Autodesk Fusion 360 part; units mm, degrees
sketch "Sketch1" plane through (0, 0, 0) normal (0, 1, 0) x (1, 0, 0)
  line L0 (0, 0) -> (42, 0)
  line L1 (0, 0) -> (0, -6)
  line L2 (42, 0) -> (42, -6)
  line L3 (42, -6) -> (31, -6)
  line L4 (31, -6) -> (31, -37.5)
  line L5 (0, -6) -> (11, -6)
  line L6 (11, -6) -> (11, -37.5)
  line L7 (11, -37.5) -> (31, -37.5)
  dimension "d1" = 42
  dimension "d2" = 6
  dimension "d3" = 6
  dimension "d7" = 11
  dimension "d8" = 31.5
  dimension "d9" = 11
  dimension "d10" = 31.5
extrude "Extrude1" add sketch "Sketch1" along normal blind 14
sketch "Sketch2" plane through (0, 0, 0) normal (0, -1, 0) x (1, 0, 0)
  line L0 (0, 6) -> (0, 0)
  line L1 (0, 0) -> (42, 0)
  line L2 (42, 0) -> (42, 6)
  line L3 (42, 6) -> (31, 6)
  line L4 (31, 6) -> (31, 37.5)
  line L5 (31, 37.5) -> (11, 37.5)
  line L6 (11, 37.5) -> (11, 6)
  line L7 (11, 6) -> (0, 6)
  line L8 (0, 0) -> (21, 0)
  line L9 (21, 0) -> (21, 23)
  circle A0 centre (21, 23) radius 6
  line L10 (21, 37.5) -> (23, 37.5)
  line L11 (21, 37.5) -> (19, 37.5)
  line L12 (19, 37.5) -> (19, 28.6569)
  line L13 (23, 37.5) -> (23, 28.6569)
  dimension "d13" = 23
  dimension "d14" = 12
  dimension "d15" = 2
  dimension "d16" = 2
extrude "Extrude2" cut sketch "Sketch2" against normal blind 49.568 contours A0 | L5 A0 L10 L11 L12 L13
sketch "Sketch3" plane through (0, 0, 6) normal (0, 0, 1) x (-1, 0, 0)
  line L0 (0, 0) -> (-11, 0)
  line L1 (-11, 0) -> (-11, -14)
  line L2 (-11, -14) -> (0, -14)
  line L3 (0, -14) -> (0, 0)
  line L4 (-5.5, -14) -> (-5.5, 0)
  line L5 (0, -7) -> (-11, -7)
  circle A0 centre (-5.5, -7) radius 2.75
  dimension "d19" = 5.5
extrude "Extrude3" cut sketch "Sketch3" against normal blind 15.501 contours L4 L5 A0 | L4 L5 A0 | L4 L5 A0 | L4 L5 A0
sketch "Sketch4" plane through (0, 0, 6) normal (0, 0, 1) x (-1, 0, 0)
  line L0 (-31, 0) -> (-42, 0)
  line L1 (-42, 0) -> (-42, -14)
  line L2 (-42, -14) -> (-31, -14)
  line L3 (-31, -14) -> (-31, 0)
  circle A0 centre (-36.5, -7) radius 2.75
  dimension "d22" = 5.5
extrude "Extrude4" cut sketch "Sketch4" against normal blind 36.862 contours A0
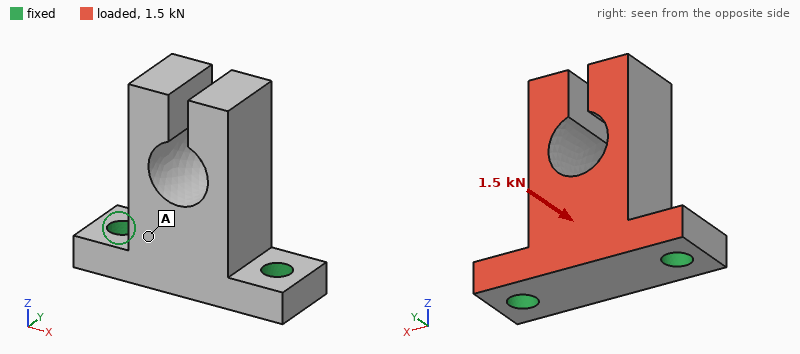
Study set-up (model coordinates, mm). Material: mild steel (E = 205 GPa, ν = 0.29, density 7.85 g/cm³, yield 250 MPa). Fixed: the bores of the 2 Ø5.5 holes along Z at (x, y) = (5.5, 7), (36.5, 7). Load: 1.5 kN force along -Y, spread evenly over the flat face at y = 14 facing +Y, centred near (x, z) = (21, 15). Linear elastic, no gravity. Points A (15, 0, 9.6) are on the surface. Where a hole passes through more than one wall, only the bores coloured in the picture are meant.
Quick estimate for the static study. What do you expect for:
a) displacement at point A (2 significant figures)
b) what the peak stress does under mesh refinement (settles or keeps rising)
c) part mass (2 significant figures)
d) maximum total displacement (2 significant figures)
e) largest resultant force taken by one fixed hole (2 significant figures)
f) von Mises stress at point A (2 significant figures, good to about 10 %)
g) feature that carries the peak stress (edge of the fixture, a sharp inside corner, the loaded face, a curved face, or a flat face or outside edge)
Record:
8.3 µm
keeps rising
78 g
34 µm
750 N
17 MPa
edge of the fixture
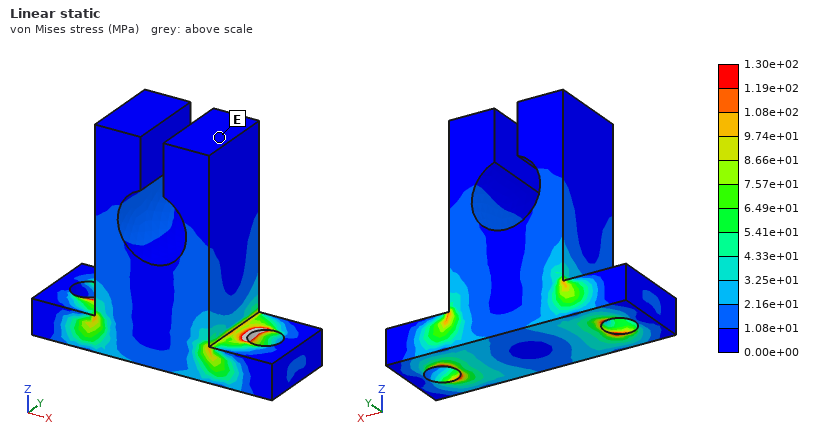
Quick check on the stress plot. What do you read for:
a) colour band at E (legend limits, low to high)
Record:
0.00e+00 to 1.08e+01 MPa
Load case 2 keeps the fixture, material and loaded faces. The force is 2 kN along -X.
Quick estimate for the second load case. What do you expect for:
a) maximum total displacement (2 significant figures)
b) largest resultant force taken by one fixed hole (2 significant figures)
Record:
35 µm
1.5 kN
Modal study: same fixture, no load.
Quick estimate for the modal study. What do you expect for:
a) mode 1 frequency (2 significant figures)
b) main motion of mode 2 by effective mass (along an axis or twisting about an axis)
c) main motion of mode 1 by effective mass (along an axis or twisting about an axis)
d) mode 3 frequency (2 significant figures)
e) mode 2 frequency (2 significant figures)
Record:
4600 Hz
along X
along Y
6100 Hz
5600 Hz
